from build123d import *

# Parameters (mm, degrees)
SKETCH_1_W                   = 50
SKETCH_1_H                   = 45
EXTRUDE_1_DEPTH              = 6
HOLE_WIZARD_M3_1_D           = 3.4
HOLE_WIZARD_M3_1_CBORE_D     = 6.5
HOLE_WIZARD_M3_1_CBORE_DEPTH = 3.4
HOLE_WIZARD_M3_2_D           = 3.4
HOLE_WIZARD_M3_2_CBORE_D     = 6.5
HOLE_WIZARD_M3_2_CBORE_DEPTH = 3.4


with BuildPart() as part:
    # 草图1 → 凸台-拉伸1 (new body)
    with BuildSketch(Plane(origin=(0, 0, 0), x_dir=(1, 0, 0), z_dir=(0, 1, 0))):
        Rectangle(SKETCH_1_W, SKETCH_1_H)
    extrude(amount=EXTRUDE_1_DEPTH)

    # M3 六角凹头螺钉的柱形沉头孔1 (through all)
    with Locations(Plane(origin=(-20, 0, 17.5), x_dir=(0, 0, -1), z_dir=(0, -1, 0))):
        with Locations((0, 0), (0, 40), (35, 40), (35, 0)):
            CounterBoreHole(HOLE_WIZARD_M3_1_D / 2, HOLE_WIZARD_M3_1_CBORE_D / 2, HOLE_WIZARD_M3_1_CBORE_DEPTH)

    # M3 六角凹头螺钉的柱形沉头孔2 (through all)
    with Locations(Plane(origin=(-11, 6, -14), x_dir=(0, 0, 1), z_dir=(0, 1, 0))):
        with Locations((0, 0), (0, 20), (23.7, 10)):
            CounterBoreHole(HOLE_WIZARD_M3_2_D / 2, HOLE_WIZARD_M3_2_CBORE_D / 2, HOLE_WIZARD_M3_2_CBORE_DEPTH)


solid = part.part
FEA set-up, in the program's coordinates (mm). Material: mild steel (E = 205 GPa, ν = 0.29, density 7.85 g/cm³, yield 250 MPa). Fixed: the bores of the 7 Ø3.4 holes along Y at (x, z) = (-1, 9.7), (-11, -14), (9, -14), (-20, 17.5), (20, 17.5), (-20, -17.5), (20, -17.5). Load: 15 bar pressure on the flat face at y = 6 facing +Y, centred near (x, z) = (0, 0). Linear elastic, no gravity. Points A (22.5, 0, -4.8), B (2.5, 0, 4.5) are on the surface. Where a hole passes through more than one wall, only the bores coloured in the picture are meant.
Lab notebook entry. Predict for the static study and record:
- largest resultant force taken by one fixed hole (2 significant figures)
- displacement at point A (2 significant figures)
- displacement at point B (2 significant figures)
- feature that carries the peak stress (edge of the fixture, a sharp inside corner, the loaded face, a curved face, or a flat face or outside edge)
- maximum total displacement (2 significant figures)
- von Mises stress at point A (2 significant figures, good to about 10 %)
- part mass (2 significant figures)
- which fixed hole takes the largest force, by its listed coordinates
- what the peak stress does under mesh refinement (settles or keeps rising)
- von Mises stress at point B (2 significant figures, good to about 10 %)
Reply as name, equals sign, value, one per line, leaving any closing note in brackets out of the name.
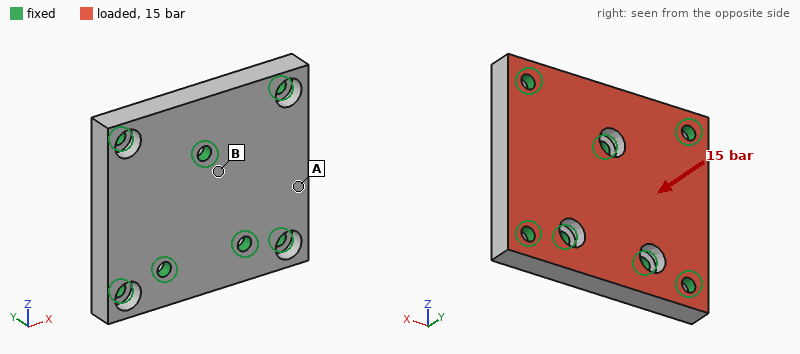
largest resultant force taken by one fixed hole = 780 N
displacement at point A = 2.4 µm
displacement at point B = 1.2 µm
feature that carries the peak stress = edge of the fixture
maximum total displacement = 3.0 µm
von Mises stress at point A = 13 MPa
part mass = 98 g
which fixed hole takes the largest force, by its listed coordinates = (-1, 9.7)
what the peak stress does under mesh refinement = keeps rising
von Mises stress at point B = 6.8 MPa
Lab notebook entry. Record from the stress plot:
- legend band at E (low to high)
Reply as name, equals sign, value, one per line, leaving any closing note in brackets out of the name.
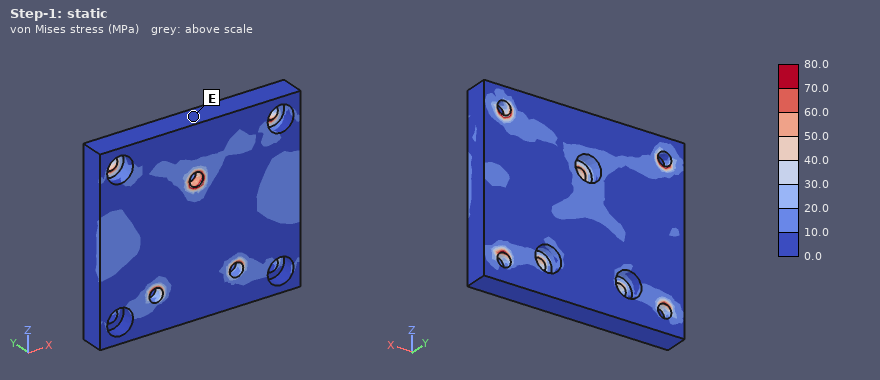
legend band at E = 0.0 to 10.0 MPa
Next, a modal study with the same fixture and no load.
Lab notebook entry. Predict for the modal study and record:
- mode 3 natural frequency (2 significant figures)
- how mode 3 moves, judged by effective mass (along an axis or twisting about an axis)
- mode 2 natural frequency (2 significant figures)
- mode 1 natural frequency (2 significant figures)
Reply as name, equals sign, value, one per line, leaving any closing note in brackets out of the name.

mode 3 natural frequency = 25 kHz
how mode 3 moves, judged by effective mass = along Y
mode 2 natural frequency = 20 kHz
mode 1 natural frequency = 19 kHz
